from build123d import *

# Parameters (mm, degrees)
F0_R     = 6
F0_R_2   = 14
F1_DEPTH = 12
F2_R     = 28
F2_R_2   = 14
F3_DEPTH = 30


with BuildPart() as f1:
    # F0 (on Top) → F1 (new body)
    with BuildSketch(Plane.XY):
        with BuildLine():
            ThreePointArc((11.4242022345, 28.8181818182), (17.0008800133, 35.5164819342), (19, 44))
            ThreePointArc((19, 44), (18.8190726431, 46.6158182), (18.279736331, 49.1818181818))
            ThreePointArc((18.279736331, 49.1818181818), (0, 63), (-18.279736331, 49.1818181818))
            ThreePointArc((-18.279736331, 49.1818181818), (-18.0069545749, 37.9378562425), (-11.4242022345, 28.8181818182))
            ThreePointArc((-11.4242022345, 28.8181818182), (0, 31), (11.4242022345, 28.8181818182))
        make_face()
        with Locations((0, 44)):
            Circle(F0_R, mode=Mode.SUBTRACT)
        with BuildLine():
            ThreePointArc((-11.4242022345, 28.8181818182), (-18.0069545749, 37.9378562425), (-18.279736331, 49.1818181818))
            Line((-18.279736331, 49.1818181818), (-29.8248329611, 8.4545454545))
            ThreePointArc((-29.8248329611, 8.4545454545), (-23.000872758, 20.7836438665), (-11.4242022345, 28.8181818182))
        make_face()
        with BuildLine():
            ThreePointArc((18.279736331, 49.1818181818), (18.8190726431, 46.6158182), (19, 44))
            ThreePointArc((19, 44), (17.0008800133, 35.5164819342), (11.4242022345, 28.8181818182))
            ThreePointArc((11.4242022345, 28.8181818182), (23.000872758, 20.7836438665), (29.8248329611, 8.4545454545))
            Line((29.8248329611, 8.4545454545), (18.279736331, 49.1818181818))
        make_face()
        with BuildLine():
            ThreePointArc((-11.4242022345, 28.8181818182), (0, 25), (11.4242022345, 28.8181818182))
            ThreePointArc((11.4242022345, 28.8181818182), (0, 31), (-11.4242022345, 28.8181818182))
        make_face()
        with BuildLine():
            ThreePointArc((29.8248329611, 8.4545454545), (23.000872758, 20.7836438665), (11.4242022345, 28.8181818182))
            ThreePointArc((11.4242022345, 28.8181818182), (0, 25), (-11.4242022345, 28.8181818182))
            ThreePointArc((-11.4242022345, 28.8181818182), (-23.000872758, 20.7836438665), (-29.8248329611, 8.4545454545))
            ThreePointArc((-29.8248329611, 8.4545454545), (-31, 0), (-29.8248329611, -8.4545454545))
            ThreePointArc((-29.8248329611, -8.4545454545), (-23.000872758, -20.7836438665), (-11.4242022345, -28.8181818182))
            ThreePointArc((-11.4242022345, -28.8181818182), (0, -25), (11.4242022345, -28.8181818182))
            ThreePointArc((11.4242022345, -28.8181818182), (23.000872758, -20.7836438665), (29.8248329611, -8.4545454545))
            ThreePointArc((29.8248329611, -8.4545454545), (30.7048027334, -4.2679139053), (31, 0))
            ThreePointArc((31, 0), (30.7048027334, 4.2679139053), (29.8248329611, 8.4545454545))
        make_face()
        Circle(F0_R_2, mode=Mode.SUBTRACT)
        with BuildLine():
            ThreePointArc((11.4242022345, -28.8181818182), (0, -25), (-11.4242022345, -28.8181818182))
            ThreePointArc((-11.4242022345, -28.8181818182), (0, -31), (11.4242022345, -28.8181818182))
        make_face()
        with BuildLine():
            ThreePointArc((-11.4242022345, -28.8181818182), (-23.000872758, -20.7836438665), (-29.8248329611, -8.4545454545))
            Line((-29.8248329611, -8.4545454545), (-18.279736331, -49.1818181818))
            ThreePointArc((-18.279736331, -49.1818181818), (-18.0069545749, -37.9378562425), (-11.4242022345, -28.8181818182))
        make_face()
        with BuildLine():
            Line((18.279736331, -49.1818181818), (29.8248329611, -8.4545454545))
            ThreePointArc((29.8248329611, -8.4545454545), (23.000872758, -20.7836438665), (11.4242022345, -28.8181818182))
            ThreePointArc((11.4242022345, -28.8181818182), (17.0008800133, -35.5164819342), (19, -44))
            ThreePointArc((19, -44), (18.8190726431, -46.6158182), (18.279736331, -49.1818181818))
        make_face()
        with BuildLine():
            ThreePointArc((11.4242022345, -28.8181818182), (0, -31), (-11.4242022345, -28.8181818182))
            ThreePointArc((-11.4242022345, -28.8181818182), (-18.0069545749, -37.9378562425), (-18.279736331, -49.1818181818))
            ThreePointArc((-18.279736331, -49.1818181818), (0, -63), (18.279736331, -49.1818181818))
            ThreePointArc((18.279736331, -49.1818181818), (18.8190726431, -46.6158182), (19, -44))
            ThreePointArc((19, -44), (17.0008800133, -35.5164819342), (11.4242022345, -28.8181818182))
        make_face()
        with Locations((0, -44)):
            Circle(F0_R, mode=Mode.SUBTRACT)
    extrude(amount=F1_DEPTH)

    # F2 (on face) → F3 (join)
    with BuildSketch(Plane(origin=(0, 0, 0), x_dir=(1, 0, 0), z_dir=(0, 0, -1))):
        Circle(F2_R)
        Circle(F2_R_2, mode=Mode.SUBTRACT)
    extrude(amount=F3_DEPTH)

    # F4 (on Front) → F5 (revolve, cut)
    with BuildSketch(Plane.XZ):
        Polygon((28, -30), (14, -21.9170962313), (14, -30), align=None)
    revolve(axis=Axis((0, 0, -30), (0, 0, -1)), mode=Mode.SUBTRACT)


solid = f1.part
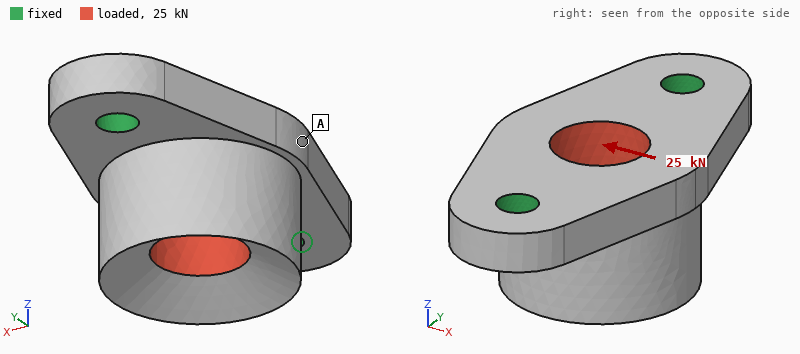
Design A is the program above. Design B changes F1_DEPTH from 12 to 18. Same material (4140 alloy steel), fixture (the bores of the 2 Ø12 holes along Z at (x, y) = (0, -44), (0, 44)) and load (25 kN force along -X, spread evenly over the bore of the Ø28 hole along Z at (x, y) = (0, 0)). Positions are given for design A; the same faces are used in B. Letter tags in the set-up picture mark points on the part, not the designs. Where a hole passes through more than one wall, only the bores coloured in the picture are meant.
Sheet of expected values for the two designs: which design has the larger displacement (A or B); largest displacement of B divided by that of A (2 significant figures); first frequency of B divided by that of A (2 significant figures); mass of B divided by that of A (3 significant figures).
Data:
A
0.48
1.4
1.27
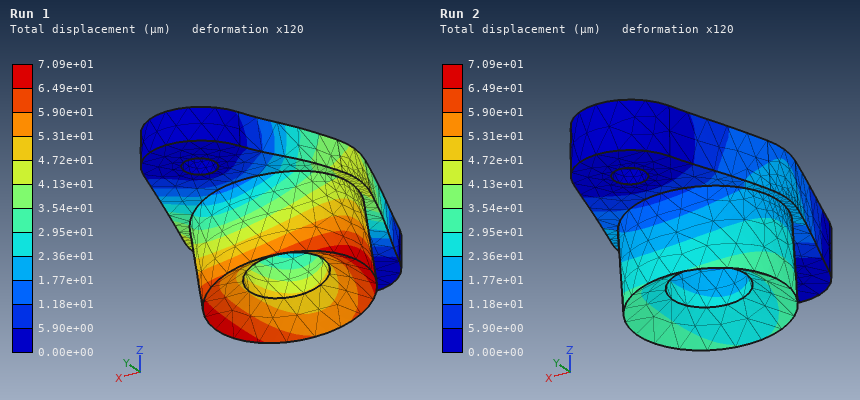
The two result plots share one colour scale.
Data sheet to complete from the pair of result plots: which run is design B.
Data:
Run 2
